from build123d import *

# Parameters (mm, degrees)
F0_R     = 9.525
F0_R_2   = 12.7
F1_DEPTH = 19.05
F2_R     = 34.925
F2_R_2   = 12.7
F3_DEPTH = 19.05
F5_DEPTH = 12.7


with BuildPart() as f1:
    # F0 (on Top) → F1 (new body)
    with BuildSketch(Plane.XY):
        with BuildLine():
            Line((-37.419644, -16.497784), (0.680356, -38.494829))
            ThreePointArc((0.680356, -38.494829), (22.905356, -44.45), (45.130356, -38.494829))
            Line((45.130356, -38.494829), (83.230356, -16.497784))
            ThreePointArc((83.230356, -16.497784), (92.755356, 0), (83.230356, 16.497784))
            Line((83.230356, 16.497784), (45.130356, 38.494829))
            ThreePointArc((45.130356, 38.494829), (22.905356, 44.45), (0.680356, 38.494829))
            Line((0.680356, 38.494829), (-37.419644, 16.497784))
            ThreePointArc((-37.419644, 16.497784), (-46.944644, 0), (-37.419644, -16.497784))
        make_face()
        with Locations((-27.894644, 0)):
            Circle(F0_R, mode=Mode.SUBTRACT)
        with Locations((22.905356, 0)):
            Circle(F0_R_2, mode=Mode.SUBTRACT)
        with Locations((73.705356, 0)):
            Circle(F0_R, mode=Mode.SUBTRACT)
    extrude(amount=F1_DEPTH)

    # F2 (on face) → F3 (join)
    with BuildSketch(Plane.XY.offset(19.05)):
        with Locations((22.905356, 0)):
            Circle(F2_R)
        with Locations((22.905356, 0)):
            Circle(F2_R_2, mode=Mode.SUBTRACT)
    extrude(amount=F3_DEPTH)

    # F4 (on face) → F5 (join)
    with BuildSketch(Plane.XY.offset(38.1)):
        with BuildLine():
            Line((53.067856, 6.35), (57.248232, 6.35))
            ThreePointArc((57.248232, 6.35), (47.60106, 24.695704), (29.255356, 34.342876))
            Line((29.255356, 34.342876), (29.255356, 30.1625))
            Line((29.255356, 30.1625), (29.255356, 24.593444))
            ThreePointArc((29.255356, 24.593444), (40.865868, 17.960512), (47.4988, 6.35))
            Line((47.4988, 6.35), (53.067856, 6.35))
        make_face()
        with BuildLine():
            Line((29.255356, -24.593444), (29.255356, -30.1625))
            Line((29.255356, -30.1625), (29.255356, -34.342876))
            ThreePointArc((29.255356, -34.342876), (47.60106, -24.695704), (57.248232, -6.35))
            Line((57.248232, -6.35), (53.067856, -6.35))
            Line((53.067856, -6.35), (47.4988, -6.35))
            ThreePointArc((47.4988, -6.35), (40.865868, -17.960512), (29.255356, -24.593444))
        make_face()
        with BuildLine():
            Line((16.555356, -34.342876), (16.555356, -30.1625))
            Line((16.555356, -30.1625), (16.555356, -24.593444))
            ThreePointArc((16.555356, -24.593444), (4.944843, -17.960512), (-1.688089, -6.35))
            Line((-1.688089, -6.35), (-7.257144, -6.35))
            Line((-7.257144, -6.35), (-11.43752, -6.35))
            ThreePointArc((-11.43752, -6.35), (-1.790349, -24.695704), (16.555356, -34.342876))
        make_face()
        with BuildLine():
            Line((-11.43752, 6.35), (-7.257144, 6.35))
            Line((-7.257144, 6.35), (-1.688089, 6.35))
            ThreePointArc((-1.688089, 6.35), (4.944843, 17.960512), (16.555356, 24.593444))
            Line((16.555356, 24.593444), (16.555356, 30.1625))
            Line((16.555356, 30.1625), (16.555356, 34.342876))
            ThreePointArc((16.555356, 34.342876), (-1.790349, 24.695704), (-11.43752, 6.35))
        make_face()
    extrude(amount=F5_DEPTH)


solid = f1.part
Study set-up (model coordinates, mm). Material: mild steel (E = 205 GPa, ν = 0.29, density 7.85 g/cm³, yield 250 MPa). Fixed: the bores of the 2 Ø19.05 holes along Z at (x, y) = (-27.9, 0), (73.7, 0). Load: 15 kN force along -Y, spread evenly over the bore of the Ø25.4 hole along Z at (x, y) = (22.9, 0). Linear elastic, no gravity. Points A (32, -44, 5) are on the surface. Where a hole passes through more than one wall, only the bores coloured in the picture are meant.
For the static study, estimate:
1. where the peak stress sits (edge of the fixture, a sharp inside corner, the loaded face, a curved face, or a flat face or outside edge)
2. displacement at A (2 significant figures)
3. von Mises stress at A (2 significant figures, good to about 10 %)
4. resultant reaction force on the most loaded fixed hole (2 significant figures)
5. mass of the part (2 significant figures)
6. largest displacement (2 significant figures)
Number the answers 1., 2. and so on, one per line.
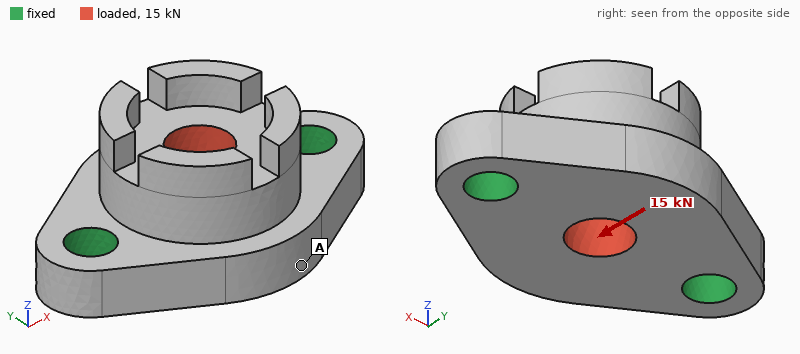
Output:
1. edge of the fixture
2. 6.7 µm
3. 7.1 MPa
4. 7.5 kN
5. 1.7 kg
6. 11 µm
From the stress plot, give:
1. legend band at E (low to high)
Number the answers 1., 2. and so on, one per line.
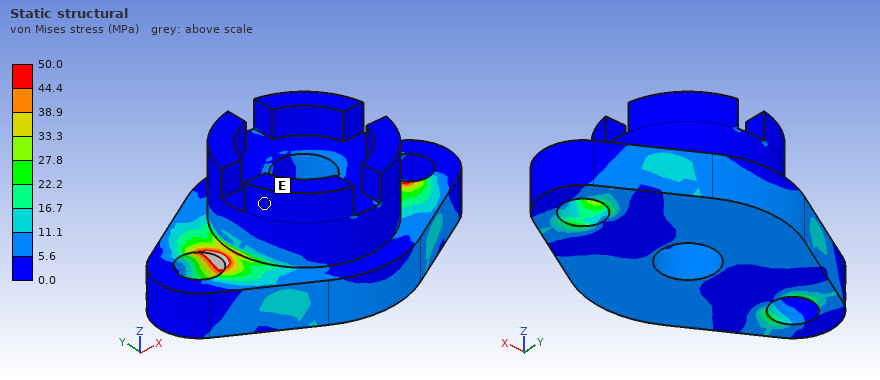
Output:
1. 0.0 to 5.6 MPa
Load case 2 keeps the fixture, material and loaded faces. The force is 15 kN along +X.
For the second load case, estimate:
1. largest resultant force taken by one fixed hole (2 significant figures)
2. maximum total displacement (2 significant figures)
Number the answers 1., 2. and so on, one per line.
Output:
1. 7.7 kN
2. 2.3 µm
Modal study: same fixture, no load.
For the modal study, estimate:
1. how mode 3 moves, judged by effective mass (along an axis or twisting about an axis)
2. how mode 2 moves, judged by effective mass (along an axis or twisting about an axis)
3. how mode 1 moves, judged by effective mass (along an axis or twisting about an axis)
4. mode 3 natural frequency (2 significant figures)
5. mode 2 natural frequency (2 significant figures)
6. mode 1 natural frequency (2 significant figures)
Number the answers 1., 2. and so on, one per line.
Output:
1. along Y
2. along Z
3. along Y
4. 11 kHz
5. 7300 Hz
6. 4700 Hz
